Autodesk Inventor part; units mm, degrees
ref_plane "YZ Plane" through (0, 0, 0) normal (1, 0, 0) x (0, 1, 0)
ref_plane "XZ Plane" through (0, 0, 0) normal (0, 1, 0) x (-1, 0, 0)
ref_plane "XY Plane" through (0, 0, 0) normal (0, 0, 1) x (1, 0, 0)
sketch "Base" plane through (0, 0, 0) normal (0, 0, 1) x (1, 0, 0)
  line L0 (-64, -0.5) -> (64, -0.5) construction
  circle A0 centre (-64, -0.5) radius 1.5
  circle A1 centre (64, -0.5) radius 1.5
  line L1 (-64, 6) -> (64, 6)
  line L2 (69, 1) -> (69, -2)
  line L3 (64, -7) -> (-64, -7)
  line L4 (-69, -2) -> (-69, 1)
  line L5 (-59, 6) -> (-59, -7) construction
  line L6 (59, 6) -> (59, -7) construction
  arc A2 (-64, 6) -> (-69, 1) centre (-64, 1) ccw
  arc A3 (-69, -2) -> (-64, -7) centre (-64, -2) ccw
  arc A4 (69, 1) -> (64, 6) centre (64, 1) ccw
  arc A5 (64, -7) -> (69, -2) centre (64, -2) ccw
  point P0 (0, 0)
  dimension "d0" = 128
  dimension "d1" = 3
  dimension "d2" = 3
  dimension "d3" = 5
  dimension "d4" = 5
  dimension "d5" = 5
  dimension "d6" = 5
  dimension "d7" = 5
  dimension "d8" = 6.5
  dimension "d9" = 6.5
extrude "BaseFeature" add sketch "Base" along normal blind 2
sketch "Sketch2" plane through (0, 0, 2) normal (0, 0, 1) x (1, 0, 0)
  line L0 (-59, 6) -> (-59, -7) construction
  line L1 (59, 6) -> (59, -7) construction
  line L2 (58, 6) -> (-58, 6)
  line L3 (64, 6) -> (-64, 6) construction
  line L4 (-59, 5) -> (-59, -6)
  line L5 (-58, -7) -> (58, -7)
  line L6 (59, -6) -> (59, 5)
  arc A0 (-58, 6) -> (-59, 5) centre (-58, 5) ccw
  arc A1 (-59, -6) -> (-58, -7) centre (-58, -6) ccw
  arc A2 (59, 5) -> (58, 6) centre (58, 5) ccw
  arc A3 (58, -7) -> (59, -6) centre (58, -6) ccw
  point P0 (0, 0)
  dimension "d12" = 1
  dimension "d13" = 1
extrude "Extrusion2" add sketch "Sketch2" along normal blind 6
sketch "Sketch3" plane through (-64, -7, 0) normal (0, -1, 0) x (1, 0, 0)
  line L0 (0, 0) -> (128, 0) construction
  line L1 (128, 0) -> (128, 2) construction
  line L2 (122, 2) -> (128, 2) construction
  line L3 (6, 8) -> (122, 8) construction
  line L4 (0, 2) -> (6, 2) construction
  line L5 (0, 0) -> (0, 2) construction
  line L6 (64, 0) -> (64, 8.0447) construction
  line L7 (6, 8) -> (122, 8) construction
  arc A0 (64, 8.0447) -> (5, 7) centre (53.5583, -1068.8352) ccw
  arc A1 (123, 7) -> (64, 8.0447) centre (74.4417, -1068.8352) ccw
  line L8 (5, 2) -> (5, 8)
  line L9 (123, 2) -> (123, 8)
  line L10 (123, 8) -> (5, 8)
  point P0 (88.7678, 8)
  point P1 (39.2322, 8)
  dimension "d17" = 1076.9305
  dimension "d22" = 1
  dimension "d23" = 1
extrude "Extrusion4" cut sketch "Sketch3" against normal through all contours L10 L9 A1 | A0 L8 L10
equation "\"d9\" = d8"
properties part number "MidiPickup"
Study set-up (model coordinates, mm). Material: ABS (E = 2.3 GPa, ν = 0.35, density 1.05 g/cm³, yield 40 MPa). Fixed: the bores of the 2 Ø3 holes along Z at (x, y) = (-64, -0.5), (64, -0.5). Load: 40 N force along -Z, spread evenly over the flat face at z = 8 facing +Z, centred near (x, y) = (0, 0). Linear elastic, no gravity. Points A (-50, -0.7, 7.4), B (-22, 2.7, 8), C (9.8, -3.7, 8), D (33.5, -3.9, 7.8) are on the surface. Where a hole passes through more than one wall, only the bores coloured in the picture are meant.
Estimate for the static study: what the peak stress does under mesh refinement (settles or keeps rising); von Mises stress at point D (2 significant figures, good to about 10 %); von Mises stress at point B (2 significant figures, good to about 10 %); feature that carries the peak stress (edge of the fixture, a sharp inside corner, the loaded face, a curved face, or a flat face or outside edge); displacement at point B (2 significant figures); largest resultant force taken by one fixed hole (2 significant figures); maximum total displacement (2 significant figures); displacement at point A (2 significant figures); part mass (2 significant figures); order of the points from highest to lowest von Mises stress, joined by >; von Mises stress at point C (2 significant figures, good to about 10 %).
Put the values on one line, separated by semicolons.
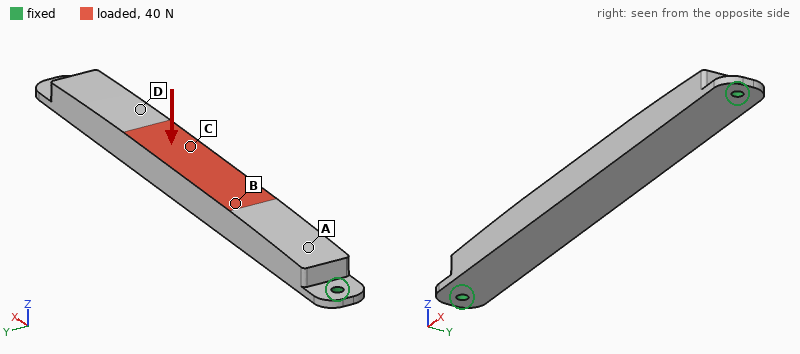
keeps rising; 2.6 MPa; 4.1 MPa; edge of the fixture; 0.53 mm; 99 N; 0.65 mm; 0.17 mm; 13 g; C > B > D > A; 5.2 MPa
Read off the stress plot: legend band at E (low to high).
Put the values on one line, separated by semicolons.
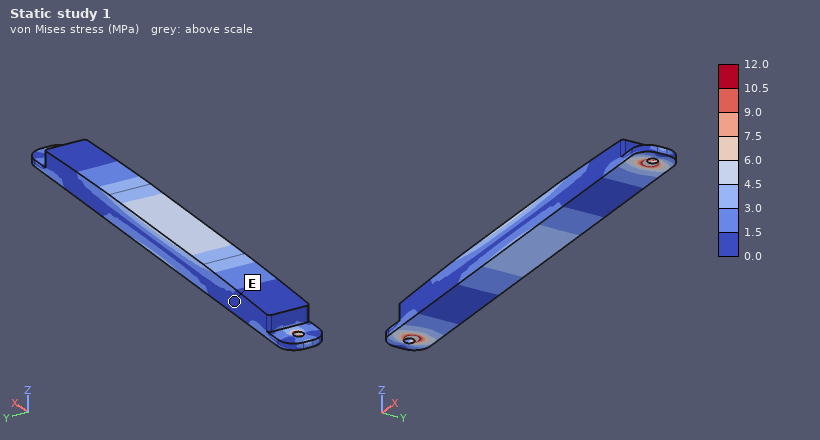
0.0 to 1.5 MPa
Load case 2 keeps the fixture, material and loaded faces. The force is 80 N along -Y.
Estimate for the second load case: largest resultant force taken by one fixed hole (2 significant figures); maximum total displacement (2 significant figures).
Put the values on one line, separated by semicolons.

40 N; 0.94 mm
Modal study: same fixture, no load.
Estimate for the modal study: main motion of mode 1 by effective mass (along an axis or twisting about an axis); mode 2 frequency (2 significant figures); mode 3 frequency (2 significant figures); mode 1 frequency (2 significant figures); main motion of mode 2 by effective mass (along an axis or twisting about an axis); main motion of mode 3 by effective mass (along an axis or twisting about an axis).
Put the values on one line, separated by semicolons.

along Z; 620 Hz; 1200 Hz; 480 Hz; along Y; twisting about X
